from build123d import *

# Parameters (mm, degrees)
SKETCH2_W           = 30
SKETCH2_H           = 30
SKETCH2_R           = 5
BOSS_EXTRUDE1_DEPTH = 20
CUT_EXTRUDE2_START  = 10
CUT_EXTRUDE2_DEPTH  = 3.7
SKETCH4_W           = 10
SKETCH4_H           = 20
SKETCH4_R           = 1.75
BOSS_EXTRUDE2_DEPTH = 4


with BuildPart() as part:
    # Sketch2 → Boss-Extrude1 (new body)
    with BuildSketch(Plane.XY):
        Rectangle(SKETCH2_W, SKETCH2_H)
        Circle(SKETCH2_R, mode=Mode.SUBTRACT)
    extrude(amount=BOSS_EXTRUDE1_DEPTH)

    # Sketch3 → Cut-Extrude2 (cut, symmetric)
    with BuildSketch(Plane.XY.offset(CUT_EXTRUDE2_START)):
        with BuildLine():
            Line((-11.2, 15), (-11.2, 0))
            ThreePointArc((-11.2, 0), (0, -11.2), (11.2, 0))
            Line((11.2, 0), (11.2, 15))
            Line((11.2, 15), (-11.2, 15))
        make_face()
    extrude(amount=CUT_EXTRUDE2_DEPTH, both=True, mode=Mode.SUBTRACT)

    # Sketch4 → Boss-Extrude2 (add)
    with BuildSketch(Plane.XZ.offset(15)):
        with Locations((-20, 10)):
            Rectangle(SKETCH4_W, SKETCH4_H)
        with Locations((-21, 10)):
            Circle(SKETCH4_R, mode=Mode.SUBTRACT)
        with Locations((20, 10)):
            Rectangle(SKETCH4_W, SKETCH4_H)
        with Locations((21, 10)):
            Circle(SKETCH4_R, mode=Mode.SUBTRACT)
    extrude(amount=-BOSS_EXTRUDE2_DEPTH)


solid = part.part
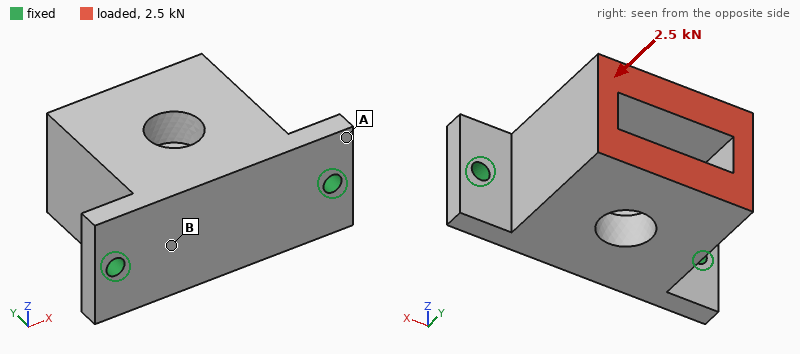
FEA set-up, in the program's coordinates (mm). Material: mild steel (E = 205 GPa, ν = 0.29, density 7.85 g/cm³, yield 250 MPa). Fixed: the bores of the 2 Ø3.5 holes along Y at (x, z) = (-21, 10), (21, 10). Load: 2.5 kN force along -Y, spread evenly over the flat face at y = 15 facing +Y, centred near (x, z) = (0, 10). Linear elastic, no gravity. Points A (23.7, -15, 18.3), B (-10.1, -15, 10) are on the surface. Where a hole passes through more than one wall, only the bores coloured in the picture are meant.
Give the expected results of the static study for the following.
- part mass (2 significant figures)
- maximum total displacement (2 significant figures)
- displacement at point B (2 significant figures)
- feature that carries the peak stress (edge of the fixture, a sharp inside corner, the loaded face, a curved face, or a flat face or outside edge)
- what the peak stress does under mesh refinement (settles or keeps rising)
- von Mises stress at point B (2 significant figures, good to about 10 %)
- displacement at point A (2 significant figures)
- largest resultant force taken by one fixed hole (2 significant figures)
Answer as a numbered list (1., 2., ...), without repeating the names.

1. 110 g
2. 6.9 µm
3. 6.0 µm
4. edge of the fixture
5. keeps rising
6. 21 MPa
7. 1.6 µm
8. 1.3 kN
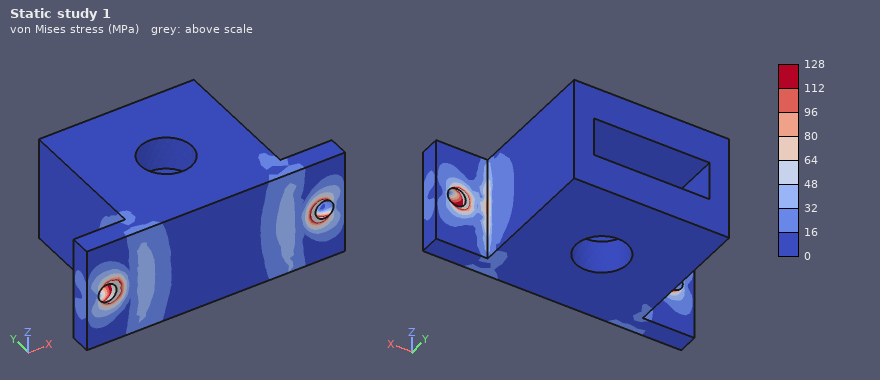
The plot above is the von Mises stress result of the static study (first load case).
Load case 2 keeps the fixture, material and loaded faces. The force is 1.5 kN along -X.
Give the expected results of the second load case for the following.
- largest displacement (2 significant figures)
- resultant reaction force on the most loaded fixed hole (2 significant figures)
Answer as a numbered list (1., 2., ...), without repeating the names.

1. 14 µm
2. 1.4 kN
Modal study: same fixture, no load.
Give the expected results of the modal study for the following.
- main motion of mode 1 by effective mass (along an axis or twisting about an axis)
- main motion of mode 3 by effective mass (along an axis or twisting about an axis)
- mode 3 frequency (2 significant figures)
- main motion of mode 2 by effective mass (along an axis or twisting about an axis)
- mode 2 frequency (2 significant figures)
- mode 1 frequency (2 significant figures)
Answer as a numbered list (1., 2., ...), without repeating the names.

1. along Z
2. along Y
3. 9700 Hz
4. along X
5. 9200 Hz
6. 2800 Hz
